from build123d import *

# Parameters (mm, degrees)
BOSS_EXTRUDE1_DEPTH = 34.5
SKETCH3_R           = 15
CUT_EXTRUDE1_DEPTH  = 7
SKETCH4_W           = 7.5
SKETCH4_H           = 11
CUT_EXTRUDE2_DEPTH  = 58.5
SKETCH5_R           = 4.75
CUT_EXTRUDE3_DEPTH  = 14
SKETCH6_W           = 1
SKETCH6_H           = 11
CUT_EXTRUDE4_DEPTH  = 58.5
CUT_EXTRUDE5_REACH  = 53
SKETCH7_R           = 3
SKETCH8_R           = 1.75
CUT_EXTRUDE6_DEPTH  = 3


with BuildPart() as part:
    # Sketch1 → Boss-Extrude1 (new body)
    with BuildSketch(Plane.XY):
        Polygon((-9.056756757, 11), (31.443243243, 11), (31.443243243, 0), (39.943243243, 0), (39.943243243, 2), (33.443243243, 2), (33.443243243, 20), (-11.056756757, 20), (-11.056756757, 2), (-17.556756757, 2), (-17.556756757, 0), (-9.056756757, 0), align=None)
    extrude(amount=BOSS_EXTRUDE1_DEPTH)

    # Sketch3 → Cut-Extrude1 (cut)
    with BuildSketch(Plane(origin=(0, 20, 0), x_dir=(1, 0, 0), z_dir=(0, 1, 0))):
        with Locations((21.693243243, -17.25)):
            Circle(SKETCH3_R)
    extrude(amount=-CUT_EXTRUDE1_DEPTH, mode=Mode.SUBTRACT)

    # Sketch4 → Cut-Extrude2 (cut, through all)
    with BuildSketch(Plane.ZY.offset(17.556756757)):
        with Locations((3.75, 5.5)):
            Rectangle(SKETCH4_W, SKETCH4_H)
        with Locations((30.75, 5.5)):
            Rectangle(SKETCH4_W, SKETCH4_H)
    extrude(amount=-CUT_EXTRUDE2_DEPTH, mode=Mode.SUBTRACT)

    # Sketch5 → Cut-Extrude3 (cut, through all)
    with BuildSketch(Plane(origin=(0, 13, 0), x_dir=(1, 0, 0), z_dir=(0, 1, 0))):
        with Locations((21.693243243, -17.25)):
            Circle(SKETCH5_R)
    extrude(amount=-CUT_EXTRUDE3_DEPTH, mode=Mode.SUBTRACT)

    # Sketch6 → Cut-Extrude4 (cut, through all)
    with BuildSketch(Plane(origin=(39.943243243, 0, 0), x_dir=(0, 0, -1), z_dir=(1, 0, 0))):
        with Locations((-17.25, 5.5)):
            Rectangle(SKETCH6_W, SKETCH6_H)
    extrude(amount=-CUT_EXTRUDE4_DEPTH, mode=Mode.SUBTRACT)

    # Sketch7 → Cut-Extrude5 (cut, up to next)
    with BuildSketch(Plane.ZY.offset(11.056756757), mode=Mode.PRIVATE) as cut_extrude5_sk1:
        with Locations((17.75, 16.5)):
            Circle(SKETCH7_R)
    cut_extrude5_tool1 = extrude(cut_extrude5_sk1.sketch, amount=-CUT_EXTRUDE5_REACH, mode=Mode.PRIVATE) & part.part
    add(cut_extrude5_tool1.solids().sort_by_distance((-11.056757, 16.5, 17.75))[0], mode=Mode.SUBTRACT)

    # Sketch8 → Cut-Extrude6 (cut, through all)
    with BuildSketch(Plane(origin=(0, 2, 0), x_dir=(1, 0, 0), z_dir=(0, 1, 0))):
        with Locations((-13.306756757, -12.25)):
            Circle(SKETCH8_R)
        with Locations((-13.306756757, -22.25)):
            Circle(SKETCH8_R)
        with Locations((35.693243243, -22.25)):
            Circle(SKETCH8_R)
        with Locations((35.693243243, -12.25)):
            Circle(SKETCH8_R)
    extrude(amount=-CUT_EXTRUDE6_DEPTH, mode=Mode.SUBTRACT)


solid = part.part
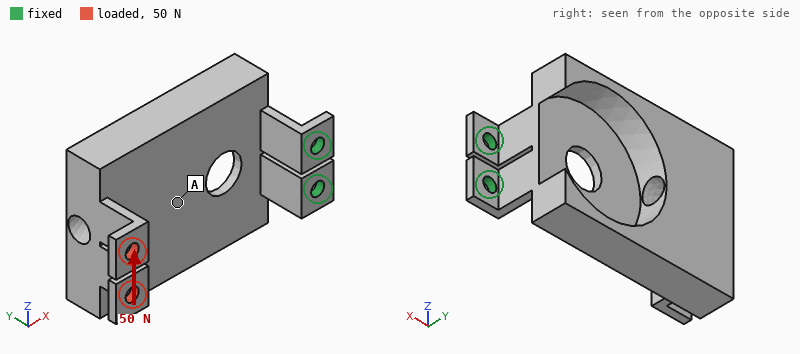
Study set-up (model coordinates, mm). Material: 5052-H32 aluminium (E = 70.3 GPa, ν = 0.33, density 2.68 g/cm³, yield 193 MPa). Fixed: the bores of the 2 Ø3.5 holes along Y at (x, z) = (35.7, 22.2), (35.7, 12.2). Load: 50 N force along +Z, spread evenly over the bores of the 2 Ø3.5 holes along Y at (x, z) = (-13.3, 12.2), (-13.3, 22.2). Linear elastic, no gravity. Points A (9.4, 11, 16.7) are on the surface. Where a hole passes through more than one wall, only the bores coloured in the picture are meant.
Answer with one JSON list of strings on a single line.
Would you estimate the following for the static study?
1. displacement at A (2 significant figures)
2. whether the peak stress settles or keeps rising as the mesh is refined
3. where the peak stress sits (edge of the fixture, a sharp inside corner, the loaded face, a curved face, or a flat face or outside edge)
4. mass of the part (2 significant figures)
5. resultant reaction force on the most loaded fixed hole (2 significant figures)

["0.21 mm", "keeps rising", "edge of the fixture", "26 g", "100 N"]
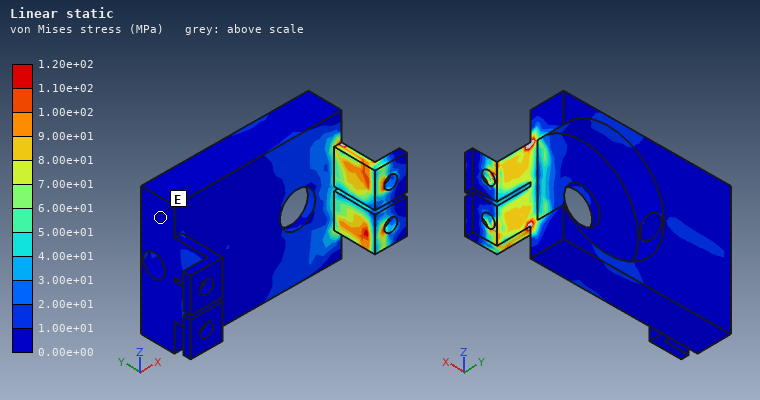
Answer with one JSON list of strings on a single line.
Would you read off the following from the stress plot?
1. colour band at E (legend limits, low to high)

["0.00e+00 to 1.00e+01 MPa"]
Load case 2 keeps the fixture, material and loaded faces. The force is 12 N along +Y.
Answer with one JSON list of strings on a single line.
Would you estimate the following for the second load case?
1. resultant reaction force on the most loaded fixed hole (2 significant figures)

["7.6 N"]
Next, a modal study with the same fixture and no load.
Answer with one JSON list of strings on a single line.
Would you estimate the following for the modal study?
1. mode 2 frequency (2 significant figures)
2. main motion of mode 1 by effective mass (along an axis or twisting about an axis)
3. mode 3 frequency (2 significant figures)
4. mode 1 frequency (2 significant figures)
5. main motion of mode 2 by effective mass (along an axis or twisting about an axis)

["520 Hz", "along Y", "2000 Hz", "250 Hz", "along Z"]
